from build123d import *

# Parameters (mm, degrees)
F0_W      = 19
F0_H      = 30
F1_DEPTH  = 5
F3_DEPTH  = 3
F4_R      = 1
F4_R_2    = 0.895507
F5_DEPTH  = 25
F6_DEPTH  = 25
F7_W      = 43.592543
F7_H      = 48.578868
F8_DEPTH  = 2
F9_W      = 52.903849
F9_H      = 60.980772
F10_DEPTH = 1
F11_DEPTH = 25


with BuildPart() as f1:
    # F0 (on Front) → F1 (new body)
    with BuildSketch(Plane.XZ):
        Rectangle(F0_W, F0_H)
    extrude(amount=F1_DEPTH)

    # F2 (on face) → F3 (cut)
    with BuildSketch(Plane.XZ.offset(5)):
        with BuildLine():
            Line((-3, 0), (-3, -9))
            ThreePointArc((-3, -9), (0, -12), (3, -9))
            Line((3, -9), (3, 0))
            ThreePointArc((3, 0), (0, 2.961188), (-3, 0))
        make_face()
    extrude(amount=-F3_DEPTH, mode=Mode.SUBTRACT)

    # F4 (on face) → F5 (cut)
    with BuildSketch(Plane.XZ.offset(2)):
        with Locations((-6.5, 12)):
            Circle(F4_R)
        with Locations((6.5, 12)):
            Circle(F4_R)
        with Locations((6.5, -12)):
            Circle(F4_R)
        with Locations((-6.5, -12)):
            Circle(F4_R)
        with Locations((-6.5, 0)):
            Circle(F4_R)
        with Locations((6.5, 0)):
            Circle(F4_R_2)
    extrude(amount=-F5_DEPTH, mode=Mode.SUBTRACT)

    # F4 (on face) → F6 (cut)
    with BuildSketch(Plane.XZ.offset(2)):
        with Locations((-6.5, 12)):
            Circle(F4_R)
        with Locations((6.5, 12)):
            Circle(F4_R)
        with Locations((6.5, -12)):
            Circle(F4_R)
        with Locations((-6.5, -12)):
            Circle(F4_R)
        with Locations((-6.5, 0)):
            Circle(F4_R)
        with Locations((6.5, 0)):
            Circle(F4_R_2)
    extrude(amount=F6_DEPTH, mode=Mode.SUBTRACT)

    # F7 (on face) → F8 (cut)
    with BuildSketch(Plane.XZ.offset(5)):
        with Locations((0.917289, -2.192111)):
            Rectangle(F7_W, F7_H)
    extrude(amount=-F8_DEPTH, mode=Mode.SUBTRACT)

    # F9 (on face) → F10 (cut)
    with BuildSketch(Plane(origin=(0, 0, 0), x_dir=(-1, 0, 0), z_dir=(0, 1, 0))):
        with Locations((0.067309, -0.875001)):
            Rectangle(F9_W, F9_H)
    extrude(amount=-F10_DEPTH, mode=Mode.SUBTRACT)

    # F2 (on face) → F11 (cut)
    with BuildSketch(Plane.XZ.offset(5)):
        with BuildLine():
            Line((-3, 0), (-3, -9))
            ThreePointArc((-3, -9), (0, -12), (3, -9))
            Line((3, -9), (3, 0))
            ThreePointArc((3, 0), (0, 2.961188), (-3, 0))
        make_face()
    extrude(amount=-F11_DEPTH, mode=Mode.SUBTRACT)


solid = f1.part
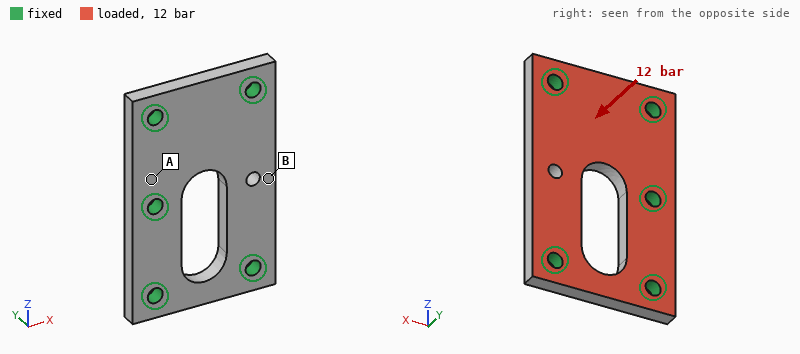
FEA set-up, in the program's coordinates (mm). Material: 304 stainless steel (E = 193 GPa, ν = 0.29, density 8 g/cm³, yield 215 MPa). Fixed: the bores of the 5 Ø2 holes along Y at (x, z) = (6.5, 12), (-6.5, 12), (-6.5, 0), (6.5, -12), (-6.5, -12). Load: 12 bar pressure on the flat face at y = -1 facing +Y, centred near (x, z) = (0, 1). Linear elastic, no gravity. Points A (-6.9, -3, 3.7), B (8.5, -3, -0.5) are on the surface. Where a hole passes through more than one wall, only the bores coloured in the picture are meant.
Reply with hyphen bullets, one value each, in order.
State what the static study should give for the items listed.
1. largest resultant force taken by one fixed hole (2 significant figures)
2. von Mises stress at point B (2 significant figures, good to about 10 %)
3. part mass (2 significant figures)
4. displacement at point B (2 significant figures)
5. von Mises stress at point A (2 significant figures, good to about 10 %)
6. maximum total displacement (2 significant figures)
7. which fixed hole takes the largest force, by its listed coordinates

- 150 N
- 42 MPa
- 7.5 g
- 7.3 µm
- 13 MPa
- 7.6 µm
- (6.5, 12)
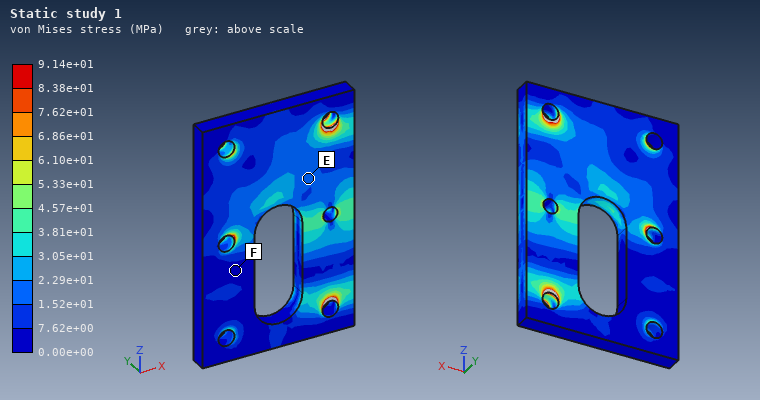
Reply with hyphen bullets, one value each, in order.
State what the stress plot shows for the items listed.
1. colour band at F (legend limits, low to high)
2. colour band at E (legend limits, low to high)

- 0.00e+00 to 7.62e+00 MPa
- 1.52e+01 to 2.29e+01 MPa
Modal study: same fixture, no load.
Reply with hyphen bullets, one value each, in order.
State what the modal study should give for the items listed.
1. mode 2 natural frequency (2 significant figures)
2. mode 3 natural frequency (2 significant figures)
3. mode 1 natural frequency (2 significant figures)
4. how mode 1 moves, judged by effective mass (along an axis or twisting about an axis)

- 40 kHz
- 45 kHz
- 20 kHz
- along Y
